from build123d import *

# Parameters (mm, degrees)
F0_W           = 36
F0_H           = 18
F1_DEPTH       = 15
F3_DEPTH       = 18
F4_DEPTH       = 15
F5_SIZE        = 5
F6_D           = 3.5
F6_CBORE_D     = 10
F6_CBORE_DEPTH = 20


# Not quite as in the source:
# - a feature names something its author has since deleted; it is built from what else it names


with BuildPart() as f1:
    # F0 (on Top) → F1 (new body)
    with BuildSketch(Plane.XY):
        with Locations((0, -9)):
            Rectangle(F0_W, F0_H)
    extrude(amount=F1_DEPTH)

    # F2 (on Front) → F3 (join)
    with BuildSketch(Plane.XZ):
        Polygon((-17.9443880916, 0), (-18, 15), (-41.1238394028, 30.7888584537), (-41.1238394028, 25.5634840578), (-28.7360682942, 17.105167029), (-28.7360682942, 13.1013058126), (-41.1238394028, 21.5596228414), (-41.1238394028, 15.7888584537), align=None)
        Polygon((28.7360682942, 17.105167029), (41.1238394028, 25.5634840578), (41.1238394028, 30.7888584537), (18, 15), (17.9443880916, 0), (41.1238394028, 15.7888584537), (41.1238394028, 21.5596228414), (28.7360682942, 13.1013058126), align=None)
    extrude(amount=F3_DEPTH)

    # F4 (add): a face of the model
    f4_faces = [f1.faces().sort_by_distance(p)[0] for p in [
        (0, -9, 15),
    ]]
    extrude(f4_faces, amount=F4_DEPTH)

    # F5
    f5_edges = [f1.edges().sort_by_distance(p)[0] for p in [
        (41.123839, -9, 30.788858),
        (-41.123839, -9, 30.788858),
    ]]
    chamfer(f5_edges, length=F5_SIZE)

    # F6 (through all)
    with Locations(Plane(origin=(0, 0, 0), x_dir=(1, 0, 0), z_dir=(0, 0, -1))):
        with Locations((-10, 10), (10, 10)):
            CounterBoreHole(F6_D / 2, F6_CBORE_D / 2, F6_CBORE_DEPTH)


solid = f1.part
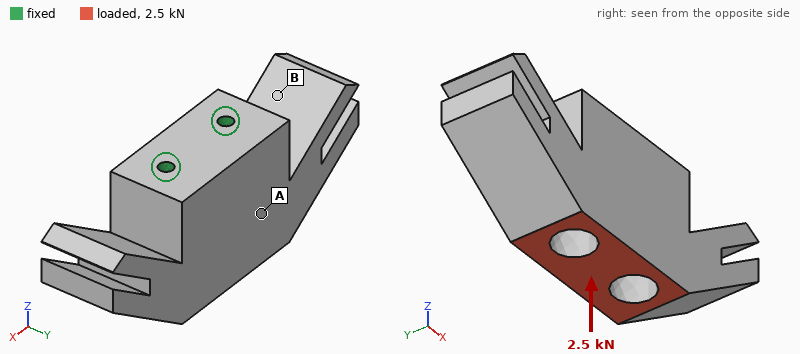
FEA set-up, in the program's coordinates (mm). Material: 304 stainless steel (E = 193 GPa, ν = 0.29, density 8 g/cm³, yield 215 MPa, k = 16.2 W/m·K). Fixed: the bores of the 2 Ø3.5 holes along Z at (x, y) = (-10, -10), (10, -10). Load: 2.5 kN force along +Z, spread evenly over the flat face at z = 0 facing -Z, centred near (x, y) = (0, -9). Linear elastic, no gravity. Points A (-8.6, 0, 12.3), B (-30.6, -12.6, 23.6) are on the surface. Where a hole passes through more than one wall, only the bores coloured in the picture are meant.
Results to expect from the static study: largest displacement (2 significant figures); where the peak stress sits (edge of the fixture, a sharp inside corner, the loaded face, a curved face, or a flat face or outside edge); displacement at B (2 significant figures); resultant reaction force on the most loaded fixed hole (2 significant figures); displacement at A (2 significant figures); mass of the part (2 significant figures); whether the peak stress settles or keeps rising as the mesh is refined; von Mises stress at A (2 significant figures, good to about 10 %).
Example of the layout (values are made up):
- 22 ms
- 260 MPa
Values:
- 1.6 µm
- edge of the fixture
- 0.75 µm
- 1.3 kN
- 1.1 µm
- 210 g
- keeps rising
- 5.5 MPa
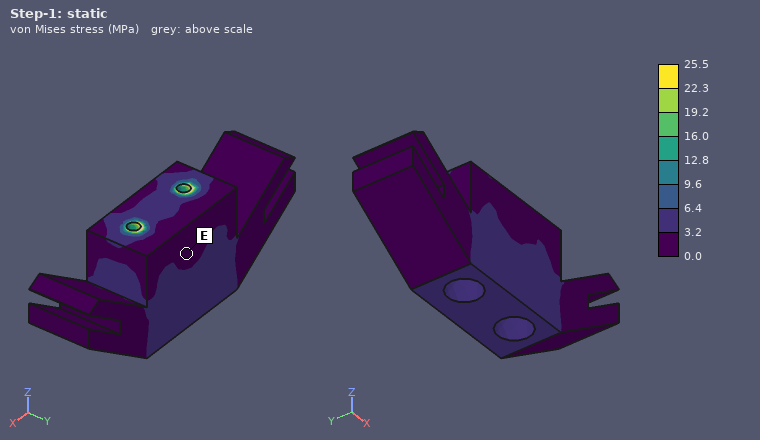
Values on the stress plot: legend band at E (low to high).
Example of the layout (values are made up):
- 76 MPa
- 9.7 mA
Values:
- 0.0 to 3.2 MPa
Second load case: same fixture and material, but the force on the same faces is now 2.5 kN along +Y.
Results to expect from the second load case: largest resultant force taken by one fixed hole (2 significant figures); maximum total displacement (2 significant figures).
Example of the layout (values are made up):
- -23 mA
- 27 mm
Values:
- 1.3 kN
- 20 µm
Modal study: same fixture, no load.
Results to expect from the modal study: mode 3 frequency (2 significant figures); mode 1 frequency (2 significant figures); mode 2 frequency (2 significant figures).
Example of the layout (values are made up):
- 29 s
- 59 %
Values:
- 7500 Hz
- 7100 Hz
- 7400 Hz
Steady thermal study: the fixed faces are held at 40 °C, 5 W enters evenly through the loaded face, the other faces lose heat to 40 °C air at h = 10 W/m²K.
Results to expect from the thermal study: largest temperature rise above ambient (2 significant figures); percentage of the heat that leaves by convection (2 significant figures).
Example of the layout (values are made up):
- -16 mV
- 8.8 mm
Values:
- 16 K
- 14 %
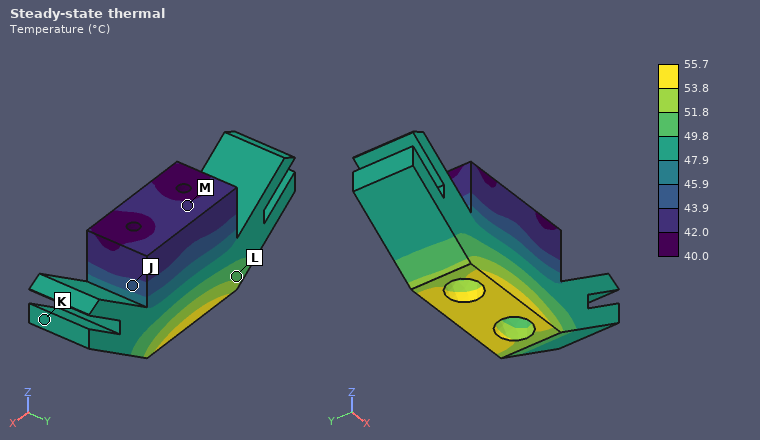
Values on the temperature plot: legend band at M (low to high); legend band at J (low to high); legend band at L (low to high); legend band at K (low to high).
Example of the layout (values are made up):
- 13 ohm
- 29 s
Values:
- 42.0 to 43.9 °C
- 43.9 to 45.9 °C
- 49.8 to 51.8 °C
- 47.9 to 49.8 °C
